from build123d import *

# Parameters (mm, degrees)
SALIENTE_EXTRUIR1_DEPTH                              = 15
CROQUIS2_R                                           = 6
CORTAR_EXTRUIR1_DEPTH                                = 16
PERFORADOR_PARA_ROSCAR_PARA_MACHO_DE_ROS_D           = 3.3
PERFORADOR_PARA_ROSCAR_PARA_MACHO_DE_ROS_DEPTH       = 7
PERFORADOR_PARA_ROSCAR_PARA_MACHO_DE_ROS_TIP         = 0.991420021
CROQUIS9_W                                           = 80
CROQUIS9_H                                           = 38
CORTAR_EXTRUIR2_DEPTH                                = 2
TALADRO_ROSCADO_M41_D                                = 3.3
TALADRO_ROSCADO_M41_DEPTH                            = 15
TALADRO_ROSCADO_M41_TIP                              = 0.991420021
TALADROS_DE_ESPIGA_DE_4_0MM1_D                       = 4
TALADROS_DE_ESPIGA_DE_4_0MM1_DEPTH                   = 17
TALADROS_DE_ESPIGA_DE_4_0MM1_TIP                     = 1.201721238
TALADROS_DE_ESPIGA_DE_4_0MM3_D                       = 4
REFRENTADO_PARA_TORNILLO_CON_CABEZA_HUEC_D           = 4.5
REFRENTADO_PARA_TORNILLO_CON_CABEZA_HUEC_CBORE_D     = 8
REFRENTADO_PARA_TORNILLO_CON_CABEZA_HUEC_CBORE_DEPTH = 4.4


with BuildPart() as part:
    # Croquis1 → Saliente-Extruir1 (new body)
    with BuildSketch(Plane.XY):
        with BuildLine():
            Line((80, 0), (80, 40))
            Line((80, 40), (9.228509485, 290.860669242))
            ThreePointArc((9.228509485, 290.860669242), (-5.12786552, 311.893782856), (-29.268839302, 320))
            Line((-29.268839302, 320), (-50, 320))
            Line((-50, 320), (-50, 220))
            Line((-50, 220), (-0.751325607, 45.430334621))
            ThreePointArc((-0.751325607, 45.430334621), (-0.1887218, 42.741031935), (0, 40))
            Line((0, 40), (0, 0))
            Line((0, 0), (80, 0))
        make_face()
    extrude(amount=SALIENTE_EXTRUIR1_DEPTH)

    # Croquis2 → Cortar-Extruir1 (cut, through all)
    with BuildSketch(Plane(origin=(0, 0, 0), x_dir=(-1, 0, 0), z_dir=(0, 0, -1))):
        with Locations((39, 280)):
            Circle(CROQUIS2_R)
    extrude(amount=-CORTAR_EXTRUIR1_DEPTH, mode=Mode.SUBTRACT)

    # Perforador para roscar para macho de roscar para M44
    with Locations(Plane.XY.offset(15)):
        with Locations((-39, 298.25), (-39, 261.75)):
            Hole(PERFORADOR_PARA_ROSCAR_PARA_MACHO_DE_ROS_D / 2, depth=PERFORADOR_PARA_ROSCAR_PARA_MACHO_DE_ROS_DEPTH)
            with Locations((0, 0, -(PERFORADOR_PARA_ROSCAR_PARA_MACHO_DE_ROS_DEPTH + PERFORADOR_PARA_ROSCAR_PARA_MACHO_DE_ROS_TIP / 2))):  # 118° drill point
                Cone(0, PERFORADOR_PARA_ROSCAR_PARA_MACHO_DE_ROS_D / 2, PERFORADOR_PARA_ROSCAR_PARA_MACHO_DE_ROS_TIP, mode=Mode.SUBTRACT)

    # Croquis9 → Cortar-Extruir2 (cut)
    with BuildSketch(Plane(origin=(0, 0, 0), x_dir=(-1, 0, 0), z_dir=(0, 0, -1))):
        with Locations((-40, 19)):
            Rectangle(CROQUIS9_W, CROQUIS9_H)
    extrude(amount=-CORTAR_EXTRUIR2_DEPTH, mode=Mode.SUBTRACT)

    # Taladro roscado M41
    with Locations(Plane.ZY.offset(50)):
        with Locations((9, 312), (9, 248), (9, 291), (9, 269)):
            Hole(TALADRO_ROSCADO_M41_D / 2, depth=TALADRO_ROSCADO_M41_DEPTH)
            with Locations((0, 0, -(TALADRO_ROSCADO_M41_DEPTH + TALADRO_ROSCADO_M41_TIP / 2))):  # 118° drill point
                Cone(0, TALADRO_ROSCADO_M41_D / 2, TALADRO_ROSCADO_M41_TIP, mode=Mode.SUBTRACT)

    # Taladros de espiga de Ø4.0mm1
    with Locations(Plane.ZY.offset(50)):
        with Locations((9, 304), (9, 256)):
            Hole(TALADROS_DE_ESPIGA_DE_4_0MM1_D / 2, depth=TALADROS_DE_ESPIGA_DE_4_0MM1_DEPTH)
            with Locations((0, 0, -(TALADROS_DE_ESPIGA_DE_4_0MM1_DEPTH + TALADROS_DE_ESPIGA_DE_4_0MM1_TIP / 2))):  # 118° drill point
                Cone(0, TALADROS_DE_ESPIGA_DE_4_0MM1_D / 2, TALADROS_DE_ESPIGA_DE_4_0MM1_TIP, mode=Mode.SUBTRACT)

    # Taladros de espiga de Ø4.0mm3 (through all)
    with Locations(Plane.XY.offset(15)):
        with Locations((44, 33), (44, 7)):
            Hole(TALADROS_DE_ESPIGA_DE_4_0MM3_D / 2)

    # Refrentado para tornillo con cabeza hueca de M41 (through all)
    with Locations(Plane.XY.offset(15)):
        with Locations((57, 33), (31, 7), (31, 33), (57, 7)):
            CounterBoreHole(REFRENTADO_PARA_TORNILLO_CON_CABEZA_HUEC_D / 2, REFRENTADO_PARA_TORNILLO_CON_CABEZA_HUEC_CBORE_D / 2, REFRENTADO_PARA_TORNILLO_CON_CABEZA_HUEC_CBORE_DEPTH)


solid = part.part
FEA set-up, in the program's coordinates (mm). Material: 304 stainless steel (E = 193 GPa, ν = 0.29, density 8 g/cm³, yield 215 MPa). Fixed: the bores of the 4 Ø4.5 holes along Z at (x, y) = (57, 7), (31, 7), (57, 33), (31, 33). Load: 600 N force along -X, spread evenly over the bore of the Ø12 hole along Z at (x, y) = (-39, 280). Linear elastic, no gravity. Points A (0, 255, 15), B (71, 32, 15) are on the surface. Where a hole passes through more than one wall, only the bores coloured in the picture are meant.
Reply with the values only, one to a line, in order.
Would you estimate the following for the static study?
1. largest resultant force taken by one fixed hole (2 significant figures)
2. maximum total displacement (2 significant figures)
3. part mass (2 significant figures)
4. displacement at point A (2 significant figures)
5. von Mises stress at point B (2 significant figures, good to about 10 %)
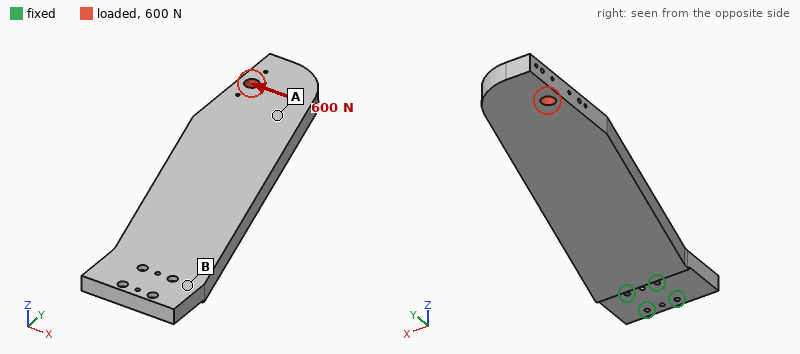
2.8 kN
56 µm
2.8 kg
39 µm
6.0 MPa
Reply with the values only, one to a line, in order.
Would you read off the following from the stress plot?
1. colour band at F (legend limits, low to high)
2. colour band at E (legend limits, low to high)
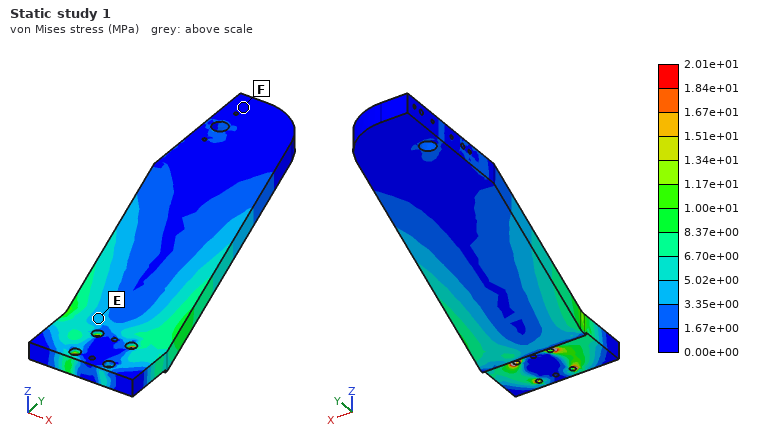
0.00e+00 to 1.67e+00 MPa
3.35e+00 to 5.02e+00 MPa
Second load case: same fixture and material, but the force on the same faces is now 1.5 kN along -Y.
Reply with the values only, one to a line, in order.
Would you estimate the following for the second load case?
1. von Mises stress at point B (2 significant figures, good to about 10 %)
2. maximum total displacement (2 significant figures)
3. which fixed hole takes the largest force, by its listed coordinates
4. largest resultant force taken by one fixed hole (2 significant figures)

4.1 MPa
50 µm
(31, 33)
2.6 kN
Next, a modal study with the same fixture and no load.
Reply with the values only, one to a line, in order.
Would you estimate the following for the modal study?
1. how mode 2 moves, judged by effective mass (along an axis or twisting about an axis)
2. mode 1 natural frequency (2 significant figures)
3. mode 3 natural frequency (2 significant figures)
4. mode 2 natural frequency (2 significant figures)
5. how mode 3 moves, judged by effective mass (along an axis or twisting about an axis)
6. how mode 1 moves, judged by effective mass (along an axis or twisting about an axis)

along X
140 Hz
830 Hz
600 Hz
along Z
along Z
